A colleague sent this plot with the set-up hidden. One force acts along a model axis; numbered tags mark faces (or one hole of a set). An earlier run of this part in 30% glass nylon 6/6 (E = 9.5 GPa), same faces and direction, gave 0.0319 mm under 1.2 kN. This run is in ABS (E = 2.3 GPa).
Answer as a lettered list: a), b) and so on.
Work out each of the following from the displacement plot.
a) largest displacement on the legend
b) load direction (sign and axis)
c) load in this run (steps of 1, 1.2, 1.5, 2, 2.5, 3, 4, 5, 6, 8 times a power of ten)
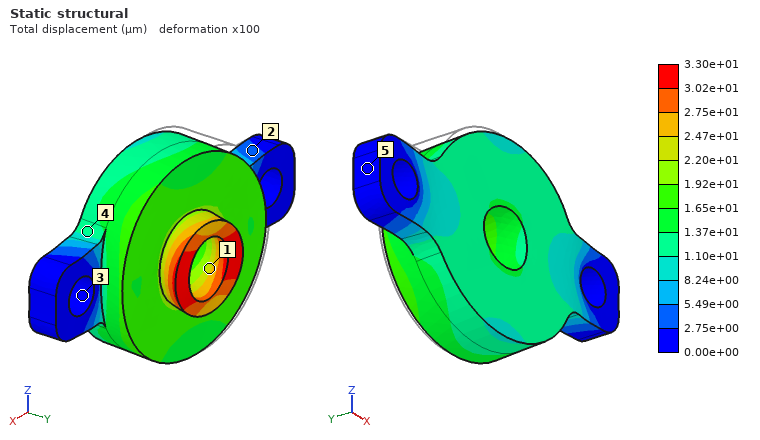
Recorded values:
a) 3.30e+01 µm
b) +X
c) 300 N
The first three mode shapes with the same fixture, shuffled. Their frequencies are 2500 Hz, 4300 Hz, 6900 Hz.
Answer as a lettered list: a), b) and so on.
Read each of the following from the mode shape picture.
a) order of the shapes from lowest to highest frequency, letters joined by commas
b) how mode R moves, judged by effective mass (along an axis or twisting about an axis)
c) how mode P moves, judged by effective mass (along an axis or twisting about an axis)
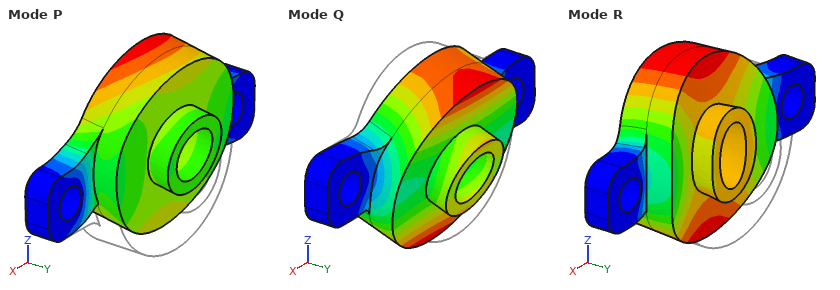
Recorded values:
a) Q, R, P
b) along Y
c) along Z
